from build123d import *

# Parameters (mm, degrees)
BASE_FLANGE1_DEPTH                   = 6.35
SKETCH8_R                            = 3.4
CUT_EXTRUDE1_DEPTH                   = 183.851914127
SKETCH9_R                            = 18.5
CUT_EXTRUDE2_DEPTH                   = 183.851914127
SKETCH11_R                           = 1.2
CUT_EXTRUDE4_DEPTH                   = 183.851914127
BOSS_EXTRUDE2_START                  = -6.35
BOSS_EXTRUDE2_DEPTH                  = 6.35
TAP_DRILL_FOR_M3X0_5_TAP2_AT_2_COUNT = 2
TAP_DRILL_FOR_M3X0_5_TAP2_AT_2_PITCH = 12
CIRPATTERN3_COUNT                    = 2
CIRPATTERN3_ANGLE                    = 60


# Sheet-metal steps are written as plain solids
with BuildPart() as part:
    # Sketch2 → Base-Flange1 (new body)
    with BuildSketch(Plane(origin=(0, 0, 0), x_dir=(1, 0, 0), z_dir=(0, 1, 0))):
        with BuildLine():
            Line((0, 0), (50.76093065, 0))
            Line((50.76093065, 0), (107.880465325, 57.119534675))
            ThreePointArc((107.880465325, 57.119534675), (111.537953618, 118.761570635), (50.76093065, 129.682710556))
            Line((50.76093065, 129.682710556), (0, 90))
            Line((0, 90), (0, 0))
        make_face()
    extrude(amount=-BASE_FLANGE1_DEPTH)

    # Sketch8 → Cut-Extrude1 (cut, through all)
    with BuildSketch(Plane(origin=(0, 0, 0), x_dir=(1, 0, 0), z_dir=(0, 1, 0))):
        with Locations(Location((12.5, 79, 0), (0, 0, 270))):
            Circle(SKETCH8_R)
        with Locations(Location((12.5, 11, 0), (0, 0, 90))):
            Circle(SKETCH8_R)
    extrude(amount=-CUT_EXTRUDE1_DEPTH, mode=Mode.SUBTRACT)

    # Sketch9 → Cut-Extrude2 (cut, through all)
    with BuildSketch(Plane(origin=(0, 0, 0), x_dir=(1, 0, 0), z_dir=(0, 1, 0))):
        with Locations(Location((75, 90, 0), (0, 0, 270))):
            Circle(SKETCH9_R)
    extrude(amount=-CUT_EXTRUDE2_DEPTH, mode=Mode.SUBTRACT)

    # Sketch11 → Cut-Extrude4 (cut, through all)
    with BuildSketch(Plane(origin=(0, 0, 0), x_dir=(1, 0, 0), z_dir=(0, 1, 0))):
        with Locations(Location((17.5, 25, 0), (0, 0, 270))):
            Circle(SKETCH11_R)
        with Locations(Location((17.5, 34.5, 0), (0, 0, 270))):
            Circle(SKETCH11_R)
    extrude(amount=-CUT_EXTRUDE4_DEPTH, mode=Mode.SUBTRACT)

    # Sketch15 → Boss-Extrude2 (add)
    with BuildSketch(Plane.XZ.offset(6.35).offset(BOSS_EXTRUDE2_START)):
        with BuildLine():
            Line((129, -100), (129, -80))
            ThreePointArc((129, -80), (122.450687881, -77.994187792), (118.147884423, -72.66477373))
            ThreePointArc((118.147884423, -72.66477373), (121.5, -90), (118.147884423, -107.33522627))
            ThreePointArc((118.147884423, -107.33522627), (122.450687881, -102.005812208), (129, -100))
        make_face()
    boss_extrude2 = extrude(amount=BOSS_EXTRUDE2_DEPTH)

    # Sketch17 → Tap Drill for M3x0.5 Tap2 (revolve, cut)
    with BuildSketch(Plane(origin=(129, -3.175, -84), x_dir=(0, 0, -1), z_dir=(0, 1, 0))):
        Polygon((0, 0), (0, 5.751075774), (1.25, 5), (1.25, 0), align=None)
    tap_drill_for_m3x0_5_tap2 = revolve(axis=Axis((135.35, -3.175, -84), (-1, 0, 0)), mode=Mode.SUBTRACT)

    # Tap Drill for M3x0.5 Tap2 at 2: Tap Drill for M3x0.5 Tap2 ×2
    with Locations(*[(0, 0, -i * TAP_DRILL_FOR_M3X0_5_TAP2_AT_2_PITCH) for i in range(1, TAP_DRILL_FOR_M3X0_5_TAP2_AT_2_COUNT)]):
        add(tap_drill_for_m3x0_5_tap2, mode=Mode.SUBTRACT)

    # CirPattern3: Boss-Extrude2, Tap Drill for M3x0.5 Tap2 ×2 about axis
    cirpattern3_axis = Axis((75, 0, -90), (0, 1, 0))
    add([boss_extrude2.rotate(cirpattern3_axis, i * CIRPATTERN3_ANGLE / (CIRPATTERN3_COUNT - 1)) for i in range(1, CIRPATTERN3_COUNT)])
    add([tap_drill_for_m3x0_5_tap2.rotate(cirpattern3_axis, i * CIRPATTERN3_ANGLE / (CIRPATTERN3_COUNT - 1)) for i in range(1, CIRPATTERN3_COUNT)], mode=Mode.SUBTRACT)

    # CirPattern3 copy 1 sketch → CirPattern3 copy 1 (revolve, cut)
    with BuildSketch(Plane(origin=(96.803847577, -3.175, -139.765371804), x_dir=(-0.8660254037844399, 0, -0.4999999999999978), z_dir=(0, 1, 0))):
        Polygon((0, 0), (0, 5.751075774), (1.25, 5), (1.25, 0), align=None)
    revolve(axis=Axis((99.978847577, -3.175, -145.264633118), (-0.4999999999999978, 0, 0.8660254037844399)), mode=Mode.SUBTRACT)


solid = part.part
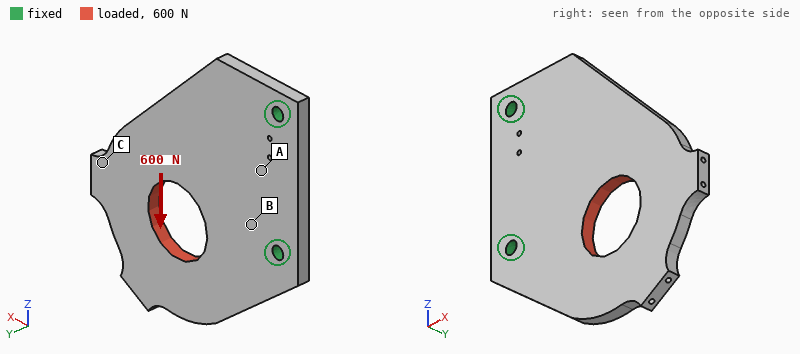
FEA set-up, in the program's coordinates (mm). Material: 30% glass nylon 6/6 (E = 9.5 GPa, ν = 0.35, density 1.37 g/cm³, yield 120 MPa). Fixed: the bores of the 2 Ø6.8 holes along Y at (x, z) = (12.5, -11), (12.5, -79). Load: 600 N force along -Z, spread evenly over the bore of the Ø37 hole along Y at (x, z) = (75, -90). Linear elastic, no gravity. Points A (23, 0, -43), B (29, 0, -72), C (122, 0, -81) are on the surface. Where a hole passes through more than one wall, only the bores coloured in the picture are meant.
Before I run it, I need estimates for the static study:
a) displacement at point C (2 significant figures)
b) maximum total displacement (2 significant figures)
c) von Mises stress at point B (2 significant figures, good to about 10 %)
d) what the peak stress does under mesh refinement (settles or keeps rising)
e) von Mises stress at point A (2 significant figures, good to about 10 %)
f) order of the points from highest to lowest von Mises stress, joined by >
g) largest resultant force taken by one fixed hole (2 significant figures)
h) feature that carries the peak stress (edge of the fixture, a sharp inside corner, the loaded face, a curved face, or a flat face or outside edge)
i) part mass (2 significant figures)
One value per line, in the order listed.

74 µm
80 µm
3.2 MPa
keeps rising
1.6 MPa
B > A > C
610 N
edge of the fixture
99 g
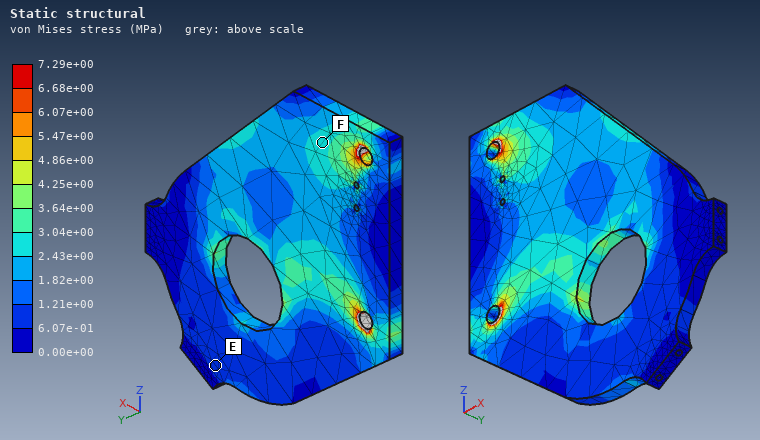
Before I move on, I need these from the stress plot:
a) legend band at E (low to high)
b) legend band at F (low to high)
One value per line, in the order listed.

6.07e-01 to 1.21e+00 MPa
2.43e+00 to 3.04e+00 MPa
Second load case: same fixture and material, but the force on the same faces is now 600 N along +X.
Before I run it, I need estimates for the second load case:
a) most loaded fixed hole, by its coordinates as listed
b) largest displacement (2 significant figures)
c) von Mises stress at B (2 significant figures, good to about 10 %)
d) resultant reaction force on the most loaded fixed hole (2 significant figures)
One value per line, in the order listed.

(12.5, -79)
52 µm
2.6 MPa
680 N
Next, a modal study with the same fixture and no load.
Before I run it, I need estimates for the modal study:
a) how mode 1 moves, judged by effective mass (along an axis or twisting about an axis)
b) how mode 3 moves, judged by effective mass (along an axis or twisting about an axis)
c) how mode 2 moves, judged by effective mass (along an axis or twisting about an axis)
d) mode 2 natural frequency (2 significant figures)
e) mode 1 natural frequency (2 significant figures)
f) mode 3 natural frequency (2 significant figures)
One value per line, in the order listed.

along Y
along Y
twisting about X
560 Hz
230 Hz
1100 Hz
